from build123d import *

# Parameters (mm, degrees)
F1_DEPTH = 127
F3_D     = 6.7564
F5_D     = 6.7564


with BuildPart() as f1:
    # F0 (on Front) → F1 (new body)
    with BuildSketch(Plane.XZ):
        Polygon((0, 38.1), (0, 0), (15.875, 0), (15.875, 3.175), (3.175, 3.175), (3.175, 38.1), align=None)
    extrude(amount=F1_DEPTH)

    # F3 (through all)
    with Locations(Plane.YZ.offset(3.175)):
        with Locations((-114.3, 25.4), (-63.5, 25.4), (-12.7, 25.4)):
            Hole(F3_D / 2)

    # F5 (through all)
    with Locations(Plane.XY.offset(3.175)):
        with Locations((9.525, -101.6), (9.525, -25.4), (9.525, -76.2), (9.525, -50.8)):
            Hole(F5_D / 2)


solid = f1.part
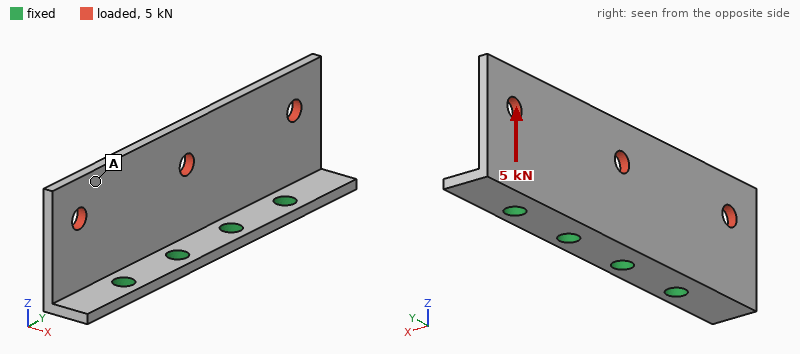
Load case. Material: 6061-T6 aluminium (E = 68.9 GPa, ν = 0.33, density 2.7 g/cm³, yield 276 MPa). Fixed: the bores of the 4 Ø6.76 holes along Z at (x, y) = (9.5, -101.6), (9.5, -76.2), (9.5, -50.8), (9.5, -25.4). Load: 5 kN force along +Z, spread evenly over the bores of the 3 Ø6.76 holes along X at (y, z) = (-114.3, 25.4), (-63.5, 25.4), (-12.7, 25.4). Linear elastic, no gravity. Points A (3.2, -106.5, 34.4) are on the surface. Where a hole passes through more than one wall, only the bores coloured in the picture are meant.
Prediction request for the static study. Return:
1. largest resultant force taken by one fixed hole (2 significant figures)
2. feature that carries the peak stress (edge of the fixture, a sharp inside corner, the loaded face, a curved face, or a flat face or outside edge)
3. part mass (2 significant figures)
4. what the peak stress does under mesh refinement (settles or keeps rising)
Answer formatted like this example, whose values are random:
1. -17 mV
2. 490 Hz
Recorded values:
1. 1.6 kN
2. edge of the fixture
3. 53 g
4. keeps rising
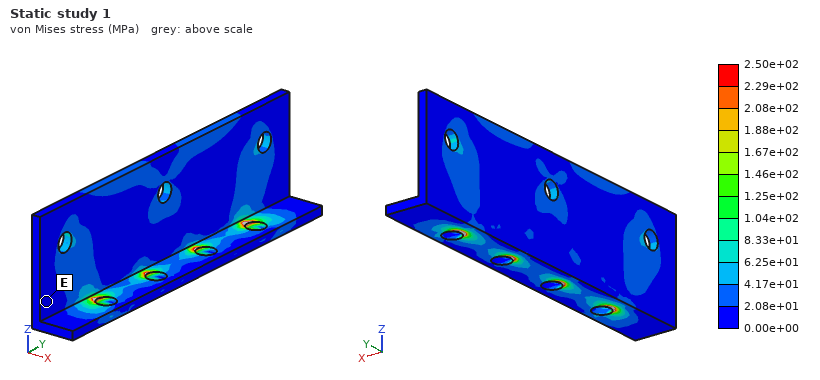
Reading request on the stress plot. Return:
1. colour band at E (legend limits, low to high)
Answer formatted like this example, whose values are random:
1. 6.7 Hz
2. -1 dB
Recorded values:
1. 0.00e+00 to 2.08e+01 MPa
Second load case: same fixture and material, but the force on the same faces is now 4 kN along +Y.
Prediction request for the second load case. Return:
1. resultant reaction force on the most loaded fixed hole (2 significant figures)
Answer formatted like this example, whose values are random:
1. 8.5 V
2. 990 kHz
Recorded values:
1. 1.4 kN
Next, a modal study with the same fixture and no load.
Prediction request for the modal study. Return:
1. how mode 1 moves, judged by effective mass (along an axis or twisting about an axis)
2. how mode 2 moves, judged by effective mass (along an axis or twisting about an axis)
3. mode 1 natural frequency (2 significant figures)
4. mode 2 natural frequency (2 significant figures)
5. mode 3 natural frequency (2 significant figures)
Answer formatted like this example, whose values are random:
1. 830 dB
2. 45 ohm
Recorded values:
1. along X
2. twisting about Z
3. 1500 Hz
4. 1800 Hz
5. 3000 Hz
